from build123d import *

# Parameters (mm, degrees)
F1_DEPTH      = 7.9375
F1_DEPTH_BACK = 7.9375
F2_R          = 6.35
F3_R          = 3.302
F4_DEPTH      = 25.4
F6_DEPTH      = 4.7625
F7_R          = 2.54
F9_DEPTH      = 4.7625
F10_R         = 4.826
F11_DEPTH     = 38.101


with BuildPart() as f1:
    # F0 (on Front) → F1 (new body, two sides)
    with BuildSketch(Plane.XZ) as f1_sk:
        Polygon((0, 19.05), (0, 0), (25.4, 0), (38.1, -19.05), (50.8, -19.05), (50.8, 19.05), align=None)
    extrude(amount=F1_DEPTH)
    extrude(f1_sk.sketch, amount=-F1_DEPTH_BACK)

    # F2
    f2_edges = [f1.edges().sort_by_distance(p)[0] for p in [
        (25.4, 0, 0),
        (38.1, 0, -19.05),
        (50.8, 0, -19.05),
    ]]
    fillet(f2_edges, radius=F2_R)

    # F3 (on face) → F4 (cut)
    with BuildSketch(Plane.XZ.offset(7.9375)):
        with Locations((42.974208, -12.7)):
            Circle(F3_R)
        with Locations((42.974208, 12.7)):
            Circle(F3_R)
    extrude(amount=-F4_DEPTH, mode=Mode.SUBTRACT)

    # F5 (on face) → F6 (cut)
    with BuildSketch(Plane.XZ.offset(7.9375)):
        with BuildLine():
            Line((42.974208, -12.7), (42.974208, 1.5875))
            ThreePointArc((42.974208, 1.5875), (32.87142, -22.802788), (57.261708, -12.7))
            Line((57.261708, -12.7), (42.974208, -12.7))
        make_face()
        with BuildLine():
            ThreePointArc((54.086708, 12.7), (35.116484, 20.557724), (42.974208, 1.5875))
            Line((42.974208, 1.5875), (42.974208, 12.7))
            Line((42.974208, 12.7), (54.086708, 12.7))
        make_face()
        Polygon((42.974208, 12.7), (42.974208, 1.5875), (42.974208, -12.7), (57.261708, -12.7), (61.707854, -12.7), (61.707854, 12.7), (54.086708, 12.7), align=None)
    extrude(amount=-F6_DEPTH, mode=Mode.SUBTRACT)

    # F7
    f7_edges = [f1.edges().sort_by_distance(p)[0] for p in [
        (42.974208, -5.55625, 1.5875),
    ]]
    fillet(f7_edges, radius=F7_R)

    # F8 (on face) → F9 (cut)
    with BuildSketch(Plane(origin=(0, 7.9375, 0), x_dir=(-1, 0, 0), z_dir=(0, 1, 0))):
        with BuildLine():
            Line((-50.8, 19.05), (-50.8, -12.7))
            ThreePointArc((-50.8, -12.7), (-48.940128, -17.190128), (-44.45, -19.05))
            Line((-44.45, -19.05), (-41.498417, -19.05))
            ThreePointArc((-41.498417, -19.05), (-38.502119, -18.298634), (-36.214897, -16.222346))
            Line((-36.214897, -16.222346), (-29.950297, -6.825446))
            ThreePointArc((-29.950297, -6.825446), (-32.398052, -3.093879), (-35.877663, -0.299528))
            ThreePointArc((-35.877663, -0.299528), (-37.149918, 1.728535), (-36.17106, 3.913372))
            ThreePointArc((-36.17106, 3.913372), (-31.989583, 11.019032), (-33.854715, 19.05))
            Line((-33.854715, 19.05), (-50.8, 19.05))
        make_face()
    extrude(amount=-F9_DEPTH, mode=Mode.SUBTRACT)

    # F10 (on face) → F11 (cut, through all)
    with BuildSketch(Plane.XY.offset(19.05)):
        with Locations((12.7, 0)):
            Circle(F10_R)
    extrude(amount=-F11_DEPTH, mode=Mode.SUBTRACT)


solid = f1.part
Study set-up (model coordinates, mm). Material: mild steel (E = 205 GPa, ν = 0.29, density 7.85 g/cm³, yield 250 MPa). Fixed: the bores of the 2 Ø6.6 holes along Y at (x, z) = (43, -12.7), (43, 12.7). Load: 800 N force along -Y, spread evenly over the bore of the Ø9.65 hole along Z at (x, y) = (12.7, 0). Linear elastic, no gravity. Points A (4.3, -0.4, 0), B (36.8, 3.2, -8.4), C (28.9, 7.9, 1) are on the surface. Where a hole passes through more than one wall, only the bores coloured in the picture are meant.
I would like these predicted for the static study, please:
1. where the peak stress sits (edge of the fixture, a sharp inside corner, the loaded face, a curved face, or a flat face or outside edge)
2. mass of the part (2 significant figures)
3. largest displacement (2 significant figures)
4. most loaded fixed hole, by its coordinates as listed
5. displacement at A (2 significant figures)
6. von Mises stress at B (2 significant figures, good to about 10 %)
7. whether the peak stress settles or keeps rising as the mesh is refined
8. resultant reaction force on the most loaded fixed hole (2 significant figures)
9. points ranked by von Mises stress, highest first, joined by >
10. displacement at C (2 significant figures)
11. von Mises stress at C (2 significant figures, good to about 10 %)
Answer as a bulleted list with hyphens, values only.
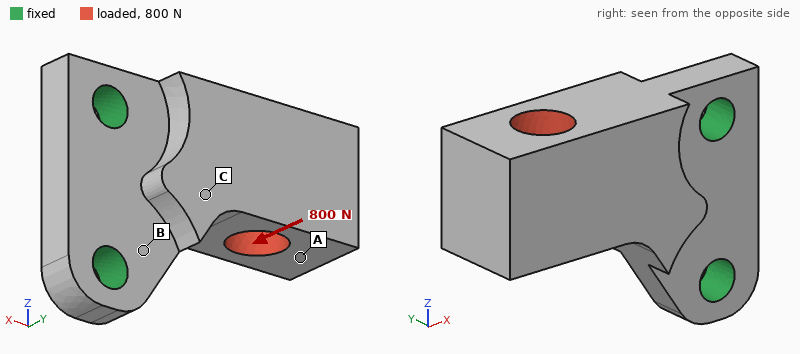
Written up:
- edge of the fixture
- 100 g
- 61 µm
- (43, 12.7)
- 52 µm
- 69 MPa
- keeps rising
- 640 N
- B > C > A
- 17 µm
- 30 MPa
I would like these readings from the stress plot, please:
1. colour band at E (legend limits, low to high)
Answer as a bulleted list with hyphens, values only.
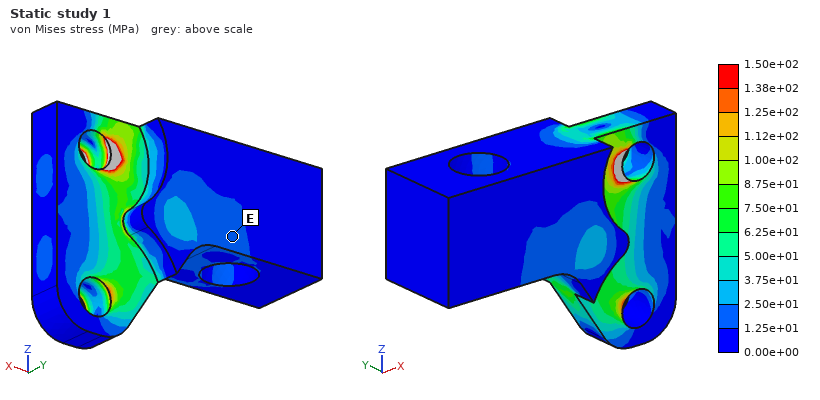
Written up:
- 1.25e+01 to 2.50e+01 MPa
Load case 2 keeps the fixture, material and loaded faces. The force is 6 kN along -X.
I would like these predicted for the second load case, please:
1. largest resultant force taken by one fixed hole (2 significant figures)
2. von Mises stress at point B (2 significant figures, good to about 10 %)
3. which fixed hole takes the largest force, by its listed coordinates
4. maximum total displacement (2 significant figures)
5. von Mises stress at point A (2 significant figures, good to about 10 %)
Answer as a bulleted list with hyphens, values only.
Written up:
- 5.1 kN
- 13 MPa
- (43, 12.7)
- 7.8 µm
- 9.1 MPa
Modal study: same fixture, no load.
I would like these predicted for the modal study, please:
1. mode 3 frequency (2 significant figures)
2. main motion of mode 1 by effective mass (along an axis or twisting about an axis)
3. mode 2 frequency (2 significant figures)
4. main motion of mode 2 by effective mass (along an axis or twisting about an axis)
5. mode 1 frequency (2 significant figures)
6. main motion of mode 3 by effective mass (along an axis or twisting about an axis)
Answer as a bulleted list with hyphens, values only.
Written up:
- 14 kHz
- along Y
- 8500 Hz
- along Z
- 2900 Hz
- twisting about X
